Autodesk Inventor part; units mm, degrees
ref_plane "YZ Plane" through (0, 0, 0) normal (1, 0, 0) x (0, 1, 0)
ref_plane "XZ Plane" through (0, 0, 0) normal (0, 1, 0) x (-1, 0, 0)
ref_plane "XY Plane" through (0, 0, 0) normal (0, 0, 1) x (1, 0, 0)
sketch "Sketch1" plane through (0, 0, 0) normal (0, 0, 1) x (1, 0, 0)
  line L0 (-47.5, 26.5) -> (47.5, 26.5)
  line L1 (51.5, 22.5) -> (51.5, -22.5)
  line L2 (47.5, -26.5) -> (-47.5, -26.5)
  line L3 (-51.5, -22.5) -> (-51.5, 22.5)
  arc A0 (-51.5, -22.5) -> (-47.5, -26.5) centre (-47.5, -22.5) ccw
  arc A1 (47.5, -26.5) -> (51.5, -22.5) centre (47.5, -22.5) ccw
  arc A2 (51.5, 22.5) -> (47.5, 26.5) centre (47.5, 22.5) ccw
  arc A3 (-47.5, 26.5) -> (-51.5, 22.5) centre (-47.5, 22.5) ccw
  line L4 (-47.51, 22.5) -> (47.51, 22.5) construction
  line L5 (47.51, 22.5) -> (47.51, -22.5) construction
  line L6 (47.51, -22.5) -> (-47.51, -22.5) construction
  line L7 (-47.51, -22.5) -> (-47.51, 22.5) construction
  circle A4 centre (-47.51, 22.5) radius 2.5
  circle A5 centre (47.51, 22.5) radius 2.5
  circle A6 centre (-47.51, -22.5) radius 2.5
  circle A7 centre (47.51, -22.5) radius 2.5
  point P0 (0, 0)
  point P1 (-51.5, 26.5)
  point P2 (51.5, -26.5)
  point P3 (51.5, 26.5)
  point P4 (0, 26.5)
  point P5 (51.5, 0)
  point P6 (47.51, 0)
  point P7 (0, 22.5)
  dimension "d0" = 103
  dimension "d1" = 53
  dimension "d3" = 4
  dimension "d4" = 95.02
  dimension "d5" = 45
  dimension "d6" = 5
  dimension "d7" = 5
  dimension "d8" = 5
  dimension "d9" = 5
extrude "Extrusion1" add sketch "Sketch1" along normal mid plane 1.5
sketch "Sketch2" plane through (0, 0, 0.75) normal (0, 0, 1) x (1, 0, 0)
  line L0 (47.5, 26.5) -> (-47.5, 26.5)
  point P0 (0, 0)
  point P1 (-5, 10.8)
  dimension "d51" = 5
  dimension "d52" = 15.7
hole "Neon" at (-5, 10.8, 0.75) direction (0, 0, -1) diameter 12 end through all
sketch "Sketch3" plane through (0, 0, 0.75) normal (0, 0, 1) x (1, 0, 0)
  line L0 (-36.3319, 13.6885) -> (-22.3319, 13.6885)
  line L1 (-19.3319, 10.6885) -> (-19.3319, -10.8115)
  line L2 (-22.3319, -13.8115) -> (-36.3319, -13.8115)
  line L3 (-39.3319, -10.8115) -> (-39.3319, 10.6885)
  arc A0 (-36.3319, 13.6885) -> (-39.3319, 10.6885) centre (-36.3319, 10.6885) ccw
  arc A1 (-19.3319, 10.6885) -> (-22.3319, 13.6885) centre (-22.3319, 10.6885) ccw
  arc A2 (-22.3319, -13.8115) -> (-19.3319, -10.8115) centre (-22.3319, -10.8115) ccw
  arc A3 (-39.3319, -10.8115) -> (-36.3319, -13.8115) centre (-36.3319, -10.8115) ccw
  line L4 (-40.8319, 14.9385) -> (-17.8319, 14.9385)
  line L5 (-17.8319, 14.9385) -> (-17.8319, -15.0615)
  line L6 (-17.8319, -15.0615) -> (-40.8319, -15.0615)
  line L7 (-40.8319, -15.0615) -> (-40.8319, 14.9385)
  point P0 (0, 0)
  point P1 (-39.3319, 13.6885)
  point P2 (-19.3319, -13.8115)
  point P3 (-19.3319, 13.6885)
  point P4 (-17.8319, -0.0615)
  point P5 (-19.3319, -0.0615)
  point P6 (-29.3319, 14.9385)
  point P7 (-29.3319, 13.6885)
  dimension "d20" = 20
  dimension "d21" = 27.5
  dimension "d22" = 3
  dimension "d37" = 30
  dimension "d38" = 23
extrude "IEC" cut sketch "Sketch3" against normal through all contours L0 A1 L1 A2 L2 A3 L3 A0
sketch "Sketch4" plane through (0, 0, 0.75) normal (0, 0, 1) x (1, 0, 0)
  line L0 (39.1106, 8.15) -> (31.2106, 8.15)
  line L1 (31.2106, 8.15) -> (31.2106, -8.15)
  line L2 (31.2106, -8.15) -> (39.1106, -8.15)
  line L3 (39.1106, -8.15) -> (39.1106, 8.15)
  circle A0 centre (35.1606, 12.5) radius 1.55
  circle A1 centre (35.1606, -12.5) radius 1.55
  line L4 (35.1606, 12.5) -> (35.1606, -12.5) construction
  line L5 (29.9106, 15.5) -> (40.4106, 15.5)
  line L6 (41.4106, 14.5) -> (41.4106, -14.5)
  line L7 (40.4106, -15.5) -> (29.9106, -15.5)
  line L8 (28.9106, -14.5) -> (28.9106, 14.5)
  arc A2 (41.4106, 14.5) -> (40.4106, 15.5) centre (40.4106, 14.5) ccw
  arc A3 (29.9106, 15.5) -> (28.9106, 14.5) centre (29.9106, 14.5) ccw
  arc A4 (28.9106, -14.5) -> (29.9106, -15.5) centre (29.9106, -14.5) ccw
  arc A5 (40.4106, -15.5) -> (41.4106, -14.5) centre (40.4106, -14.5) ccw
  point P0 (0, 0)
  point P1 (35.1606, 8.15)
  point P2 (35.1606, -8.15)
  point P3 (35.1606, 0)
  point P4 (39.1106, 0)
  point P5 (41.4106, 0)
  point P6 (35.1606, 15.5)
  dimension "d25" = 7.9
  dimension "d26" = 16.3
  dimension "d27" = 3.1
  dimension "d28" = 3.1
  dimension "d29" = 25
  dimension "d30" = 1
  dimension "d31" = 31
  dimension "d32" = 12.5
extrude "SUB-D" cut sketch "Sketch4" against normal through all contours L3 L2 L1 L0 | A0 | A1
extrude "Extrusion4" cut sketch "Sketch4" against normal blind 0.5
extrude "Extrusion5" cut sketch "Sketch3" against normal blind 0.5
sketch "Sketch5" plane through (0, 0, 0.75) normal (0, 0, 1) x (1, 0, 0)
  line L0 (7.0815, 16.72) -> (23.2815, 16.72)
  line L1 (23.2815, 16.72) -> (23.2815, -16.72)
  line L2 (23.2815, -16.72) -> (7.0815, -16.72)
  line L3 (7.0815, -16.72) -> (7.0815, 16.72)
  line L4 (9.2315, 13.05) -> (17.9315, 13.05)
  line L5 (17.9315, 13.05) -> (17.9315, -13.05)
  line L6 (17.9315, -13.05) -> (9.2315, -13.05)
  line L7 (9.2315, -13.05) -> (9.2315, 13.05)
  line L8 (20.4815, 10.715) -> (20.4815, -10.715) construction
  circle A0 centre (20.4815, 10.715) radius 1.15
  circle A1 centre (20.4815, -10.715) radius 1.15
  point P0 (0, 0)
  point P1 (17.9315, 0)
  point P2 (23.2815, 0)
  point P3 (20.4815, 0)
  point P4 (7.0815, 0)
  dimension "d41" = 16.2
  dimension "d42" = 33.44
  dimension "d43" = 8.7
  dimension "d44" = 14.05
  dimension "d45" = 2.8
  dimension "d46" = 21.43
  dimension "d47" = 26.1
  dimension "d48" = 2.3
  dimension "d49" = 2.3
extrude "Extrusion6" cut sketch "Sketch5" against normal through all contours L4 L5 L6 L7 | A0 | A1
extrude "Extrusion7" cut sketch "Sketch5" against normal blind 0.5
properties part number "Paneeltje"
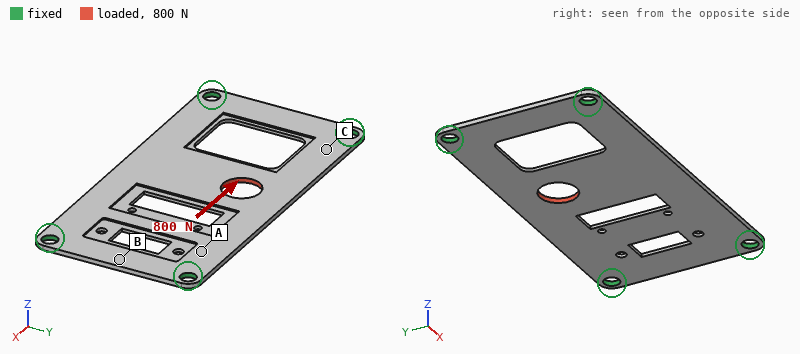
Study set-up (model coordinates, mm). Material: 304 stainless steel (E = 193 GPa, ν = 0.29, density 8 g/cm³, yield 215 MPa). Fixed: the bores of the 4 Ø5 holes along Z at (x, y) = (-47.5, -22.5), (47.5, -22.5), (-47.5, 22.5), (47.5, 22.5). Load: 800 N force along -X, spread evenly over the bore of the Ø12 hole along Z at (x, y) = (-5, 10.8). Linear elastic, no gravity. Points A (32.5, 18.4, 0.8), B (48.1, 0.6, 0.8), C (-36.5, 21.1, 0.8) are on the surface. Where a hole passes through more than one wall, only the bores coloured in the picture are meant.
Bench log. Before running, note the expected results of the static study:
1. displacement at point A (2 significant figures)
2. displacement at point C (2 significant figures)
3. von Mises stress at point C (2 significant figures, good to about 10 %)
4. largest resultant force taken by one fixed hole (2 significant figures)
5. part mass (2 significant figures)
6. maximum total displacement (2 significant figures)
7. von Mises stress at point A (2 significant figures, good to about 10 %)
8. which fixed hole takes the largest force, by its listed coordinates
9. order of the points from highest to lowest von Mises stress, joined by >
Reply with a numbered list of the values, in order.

1. 1.5 µm
2. 1.0 µm
3. 18 MPa
4. 310 N
5. 49 g
6. 5.7 µm
7. 11 MPa
8. (-47.5, 22.5)
9. C > A > B
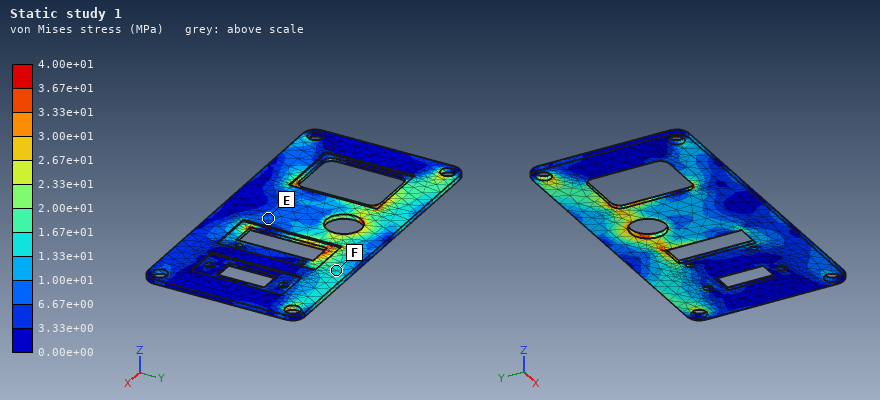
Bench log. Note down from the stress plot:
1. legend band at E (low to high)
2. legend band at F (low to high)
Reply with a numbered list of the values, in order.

1. 6.67e+00 to 1.00e+01 MPa
2. 1.33e+01 to 1.67e+01 MPa
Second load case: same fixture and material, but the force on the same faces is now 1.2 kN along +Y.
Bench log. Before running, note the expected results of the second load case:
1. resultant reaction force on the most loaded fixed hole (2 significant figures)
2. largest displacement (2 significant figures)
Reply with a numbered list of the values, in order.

1. 500 N
2. 36 µm
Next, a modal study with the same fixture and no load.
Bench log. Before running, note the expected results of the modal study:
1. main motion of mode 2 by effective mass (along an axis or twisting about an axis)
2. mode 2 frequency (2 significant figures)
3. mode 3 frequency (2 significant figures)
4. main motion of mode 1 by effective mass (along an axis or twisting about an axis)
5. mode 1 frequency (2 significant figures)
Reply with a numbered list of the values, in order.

1. twisting about X
2. 1200 Hz
3. 2000 Hz
4. along Z
5. 740 Hz
